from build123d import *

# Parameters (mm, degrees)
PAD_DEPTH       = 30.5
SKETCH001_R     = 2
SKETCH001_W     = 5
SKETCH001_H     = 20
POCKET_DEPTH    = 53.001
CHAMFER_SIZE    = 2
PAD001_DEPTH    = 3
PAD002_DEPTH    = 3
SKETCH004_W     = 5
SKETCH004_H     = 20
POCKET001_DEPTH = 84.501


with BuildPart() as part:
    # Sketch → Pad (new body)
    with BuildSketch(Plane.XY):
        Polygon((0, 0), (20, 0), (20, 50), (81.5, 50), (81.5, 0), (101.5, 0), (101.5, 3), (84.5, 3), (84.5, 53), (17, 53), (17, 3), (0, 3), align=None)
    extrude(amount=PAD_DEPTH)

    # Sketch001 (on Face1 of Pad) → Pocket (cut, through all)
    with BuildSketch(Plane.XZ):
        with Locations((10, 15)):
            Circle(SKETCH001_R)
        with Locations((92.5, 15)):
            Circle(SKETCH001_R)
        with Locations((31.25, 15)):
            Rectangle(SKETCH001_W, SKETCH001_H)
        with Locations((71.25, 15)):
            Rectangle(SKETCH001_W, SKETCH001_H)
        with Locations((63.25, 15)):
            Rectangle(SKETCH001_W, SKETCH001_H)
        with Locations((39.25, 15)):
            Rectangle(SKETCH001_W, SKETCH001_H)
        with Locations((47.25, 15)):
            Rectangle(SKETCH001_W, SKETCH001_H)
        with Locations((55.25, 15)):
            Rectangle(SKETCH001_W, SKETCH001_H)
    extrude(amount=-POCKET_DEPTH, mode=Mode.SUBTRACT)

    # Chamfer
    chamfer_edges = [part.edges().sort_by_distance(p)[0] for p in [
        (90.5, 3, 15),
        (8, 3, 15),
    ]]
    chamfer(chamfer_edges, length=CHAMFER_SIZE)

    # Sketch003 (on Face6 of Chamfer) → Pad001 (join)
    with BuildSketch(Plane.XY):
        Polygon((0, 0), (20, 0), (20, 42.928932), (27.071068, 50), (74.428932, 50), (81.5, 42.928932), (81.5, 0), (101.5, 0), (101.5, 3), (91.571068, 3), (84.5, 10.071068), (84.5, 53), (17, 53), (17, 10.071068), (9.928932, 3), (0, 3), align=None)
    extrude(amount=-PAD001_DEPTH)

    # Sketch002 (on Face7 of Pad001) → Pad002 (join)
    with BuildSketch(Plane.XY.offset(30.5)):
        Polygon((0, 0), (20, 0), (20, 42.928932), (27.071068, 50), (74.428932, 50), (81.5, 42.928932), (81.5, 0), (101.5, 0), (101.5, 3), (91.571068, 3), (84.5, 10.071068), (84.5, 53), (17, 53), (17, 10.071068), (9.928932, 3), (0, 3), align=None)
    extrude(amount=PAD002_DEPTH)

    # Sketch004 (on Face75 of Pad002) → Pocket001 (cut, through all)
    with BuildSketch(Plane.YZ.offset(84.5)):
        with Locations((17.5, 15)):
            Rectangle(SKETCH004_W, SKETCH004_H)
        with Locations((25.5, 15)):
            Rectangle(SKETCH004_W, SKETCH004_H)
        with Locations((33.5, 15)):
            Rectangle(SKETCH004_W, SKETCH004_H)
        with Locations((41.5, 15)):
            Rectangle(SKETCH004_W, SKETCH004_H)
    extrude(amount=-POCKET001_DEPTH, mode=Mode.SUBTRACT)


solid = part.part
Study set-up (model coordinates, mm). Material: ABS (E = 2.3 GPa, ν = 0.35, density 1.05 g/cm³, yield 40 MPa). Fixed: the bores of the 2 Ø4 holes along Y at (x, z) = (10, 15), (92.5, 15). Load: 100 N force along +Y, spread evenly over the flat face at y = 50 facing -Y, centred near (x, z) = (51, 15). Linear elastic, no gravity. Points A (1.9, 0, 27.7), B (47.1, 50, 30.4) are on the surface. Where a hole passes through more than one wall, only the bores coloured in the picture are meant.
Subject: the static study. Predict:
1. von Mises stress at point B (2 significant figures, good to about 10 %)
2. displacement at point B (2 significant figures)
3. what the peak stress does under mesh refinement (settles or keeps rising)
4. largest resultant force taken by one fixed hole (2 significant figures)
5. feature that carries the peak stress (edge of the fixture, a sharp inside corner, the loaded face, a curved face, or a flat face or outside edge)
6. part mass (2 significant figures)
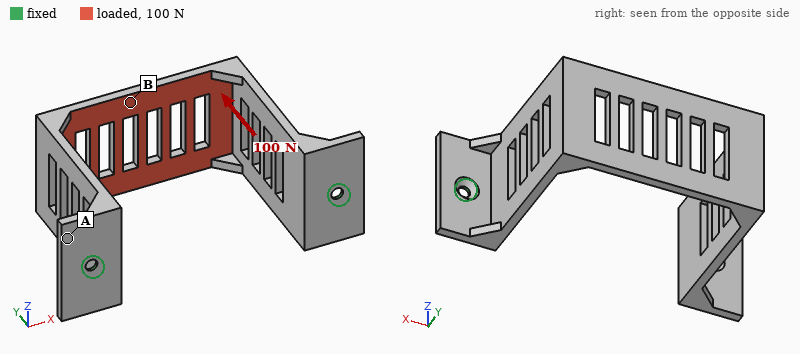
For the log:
11 MPa
1.2 mm
keeps rising
53 N
edge of the fixture
19 g
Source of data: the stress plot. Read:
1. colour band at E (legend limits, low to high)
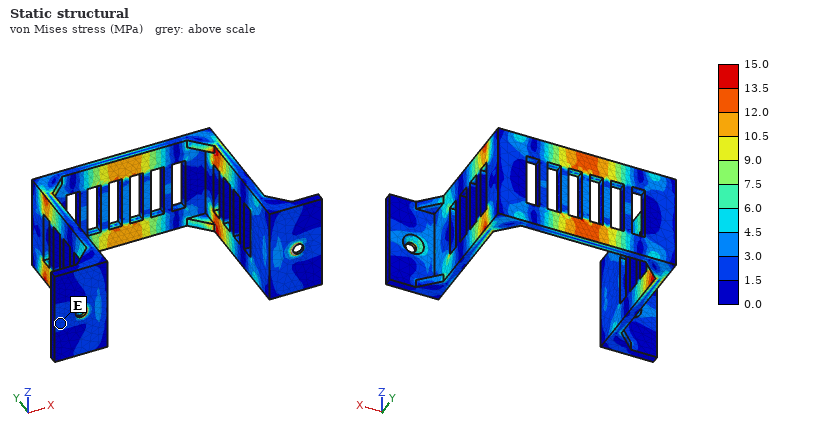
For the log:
1.5 to 3.0 MPa
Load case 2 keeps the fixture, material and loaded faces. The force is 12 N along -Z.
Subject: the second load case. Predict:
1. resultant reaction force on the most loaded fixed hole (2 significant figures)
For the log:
6.1 N
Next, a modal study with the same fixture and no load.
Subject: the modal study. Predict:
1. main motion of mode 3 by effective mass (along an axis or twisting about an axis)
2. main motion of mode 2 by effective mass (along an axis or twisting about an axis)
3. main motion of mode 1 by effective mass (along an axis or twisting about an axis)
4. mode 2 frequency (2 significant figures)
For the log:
twisting about Y
along X
along Z
190 Hz
